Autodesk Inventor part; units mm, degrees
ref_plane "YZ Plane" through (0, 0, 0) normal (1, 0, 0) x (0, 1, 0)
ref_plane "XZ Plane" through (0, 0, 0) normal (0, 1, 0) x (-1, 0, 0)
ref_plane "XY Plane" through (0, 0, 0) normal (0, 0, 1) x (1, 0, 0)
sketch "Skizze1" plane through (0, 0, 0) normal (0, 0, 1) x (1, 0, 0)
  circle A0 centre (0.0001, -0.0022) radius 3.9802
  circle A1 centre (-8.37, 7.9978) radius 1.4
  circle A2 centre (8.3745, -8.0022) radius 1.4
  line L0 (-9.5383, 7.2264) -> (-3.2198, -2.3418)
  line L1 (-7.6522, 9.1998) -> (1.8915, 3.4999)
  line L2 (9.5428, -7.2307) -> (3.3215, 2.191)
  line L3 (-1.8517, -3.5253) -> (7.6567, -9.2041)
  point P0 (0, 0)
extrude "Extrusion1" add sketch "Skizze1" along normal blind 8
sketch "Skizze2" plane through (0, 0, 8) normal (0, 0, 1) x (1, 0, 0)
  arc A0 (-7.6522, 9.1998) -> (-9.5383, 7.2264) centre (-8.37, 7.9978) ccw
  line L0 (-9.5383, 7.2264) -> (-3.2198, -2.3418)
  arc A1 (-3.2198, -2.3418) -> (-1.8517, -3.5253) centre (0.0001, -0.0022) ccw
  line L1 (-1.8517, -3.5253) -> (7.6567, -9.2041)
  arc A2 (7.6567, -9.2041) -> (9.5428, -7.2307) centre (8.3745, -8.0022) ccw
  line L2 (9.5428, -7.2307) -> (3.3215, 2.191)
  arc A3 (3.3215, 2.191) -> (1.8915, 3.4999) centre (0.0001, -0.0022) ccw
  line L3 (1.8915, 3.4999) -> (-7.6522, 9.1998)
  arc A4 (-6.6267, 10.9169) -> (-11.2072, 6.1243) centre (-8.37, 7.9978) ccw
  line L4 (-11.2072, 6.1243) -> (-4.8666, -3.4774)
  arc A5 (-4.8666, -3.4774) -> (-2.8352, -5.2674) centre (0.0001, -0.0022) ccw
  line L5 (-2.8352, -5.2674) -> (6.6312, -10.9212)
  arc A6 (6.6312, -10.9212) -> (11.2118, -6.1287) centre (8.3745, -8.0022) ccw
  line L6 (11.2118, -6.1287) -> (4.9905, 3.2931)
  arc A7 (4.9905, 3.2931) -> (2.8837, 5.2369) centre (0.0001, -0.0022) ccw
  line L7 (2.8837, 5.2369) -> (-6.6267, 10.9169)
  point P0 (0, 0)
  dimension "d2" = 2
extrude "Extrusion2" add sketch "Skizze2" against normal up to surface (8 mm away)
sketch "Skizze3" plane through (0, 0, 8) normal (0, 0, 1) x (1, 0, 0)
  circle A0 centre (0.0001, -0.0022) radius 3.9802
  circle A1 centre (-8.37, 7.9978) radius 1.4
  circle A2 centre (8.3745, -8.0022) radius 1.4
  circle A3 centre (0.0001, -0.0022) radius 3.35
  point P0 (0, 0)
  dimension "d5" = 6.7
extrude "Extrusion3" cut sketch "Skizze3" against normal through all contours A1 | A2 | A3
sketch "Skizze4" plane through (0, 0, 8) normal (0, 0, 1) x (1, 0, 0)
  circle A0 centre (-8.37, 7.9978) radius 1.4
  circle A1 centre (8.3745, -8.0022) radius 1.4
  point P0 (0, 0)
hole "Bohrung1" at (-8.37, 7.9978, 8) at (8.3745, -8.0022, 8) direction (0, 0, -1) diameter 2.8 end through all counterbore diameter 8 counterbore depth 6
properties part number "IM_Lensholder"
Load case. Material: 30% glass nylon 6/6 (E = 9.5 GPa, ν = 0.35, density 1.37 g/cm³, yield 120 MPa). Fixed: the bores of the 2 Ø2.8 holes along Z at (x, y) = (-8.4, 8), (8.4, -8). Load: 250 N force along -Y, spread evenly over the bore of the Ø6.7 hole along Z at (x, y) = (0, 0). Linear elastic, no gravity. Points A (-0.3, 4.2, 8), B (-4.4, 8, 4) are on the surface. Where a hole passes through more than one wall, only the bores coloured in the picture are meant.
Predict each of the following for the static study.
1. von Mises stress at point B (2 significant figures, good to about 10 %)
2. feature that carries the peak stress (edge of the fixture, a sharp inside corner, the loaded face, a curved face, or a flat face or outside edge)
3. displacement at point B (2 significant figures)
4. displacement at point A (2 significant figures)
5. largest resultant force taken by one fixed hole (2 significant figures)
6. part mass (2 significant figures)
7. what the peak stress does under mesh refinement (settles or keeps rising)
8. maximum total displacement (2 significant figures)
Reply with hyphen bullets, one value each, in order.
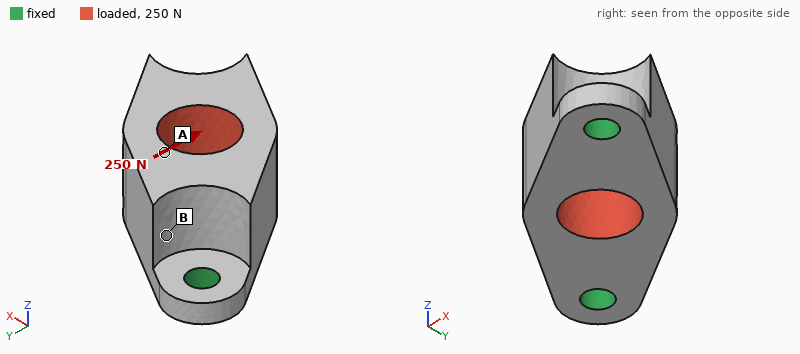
- 11 MPa
- edge of the fixture
- 40 µm
- 72 µm
- 130 N
- 1.7 g
- keeps rising
- 84 µm
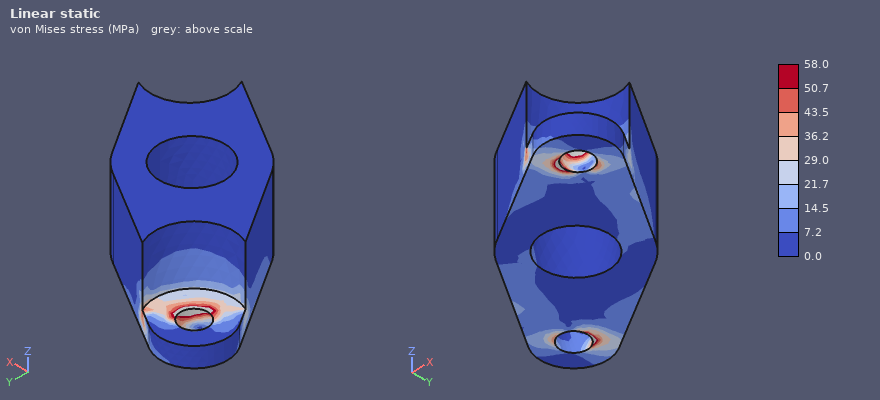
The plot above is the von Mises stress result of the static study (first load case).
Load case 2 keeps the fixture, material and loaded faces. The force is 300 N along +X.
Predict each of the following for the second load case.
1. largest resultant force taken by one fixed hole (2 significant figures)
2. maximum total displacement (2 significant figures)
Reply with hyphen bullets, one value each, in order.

- 150 N
- 97 µm
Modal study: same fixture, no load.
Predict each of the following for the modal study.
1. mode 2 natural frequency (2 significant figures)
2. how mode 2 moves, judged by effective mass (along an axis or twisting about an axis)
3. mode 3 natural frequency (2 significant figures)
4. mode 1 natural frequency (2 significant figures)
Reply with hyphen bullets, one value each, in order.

- 13 kHz
- along Z
- 21 kHz
- 6600 Hz
